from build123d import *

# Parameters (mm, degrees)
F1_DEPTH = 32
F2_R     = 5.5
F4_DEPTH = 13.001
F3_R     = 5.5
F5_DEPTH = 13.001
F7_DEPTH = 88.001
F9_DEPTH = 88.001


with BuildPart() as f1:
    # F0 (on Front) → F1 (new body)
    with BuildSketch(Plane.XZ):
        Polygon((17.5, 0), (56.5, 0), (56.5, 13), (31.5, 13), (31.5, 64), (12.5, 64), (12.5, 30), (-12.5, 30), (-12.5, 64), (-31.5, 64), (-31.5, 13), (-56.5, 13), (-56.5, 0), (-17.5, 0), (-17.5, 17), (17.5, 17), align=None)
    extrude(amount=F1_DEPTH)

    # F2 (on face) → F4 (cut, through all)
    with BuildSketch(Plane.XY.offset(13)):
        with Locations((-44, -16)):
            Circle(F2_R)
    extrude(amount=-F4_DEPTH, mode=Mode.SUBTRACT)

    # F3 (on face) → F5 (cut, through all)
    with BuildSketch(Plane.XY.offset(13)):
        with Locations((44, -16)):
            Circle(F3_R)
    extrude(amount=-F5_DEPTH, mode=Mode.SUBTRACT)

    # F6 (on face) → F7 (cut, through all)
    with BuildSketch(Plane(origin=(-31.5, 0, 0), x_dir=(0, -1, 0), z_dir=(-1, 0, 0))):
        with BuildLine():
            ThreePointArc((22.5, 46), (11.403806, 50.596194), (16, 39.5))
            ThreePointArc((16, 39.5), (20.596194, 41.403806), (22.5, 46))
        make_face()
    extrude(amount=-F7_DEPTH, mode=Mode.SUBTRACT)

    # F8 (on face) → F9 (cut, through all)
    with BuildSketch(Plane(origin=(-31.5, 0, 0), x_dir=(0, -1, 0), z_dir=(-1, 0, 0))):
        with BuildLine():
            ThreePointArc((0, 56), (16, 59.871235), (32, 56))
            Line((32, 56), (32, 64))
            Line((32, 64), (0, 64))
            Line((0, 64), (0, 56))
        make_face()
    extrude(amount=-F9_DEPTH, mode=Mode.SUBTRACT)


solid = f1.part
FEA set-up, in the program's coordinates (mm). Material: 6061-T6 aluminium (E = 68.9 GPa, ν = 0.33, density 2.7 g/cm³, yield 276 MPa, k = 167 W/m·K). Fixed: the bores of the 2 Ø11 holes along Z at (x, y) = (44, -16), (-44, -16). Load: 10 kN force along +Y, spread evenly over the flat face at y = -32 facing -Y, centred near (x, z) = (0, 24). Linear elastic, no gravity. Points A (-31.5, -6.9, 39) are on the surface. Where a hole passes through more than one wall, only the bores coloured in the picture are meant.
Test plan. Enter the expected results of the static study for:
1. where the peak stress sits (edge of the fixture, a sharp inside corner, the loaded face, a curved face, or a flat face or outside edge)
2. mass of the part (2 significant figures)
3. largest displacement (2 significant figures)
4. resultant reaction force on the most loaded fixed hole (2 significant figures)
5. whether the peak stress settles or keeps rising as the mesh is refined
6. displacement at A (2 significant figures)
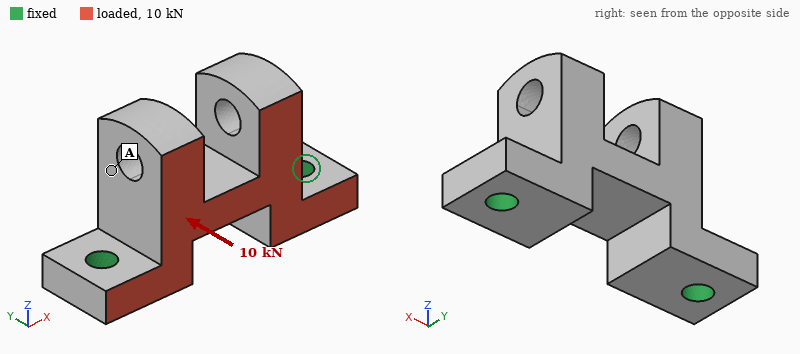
edge of the fixture
240 g
0.16 mm
5.0 kN
keeps rising
0.098 mm
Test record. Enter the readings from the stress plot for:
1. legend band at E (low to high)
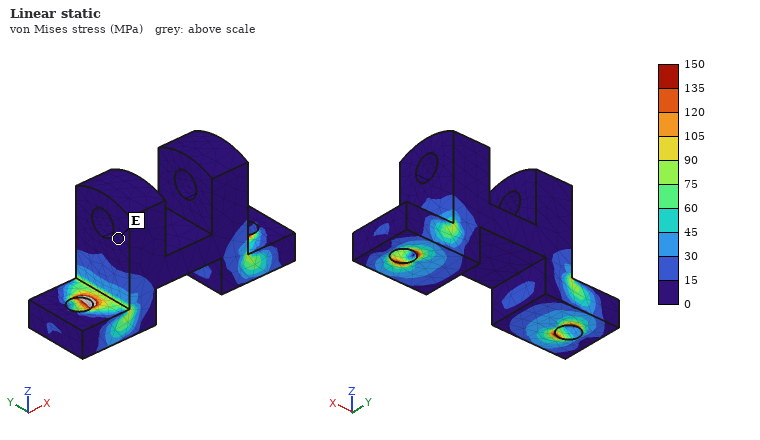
0 to 15 MPa
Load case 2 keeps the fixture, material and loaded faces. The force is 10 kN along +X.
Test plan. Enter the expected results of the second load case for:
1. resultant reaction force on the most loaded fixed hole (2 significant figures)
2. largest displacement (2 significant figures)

5.6 kN
53 µm
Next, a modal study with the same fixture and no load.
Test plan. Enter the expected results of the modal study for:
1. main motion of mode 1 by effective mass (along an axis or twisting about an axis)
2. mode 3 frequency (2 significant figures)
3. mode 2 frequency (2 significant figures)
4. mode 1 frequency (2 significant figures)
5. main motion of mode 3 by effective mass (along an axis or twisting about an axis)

along Y
6600 Hz
5300 Hz
3100 Hz
along X
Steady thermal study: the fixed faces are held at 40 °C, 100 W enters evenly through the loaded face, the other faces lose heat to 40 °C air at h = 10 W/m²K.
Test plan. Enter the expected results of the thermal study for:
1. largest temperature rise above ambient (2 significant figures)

20 K
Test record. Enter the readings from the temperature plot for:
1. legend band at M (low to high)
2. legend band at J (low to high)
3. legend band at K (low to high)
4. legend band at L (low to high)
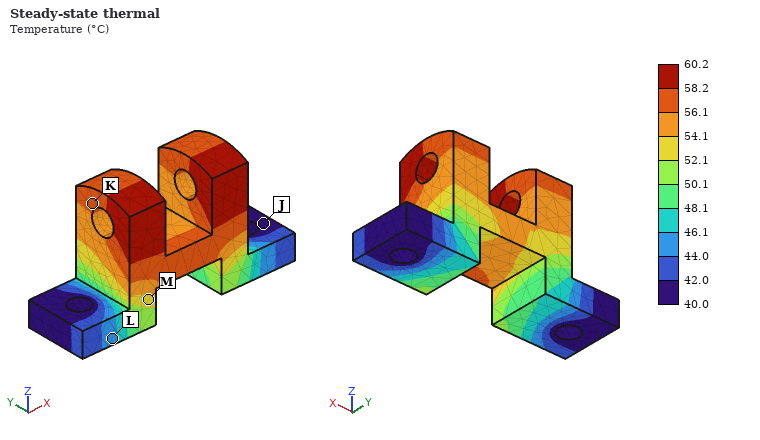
52.1 to 54.1 °C
40.0 to 42.0 °C
56.1 to 58.2 °C
44.0 to 46.1 °C
